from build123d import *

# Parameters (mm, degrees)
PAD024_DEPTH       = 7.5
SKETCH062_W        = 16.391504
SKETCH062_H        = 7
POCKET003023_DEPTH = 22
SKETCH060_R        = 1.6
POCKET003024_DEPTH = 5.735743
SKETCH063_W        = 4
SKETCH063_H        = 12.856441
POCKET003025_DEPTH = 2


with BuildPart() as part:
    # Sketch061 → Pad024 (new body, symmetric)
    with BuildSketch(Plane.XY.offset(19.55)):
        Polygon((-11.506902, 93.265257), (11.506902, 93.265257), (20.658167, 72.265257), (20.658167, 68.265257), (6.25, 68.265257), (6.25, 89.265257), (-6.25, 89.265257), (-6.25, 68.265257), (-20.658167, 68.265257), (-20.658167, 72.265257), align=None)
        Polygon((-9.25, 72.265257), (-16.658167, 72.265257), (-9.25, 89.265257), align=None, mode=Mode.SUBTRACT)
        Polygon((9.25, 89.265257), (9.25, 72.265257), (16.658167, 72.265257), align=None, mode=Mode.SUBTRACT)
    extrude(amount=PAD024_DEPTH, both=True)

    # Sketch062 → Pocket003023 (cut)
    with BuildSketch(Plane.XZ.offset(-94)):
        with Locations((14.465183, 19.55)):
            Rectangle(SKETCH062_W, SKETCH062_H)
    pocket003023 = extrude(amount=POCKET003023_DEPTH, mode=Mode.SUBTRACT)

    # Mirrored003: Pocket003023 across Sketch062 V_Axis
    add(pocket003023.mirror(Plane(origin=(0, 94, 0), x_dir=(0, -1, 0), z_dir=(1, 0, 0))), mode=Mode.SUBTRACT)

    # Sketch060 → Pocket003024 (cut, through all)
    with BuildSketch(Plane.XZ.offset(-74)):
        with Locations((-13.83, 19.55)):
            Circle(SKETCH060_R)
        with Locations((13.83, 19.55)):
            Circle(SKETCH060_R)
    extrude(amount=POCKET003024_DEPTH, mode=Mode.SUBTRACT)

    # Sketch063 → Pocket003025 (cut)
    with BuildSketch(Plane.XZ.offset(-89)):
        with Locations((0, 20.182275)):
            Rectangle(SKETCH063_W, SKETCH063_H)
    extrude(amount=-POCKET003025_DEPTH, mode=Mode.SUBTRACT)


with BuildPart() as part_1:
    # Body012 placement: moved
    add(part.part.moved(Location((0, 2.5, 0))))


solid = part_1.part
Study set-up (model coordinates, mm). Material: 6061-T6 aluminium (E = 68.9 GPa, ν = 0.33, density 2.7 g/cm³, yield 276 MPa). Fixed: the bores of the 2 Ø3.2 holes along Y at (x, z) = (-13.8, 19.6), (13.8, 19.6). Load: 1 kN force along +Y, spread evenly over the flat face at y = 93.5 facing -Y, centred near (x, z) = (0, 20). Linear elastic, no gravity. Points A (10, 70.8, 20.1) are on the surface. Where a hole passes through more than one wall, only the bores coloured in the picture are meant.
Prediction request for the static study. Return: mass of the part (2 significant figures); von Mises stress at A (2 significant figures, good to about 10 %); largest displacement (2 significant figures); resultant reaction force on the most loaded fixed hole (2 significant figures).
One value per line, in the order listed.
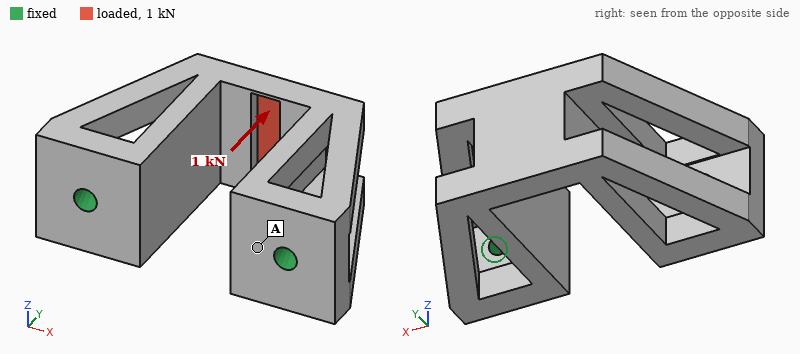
12 g
24 MPa
32 µm
530 N
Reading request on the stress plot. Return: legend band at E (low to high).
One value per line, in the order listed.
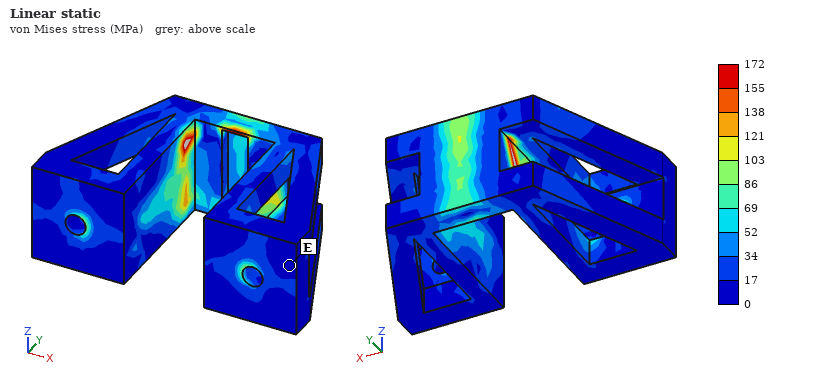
0 to 17 MPa
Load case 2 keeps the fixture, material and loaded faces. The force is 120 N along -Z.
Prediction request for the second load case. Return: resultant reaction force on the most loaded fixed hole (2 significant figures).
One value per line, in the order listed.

60 N
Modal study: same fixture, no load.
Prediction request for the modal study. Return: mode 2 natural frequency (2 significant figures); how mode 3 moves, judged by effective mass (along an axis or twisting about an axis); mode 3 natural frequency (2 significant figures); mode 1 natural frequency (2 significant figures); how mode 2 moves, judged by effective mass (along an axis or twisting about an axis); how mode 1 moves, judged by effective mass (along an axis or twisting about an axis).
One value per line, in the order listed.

7200 Hz
twisting about Y
8700 Hz
4800 Hz
along X
along Z
